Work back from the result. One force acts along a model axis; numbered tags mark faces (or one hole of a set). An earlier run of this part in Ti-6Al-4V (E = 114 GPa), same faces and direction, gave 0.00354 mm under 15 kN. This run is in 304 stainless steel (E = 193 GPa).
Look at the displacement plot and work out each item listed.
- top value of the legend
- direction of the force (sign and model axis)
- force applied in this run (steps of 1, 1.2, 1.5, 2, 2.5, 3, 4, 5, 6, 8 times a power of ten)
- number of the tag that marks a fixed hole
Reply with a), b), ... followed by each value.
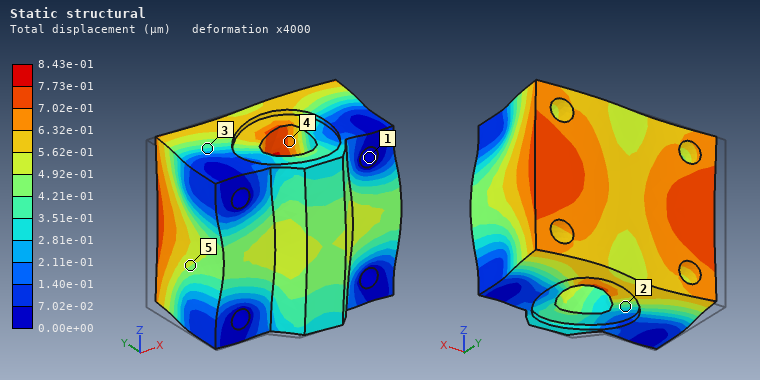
a) 8.43e-01 µm
b) +X
c) 6 kN
d) 1
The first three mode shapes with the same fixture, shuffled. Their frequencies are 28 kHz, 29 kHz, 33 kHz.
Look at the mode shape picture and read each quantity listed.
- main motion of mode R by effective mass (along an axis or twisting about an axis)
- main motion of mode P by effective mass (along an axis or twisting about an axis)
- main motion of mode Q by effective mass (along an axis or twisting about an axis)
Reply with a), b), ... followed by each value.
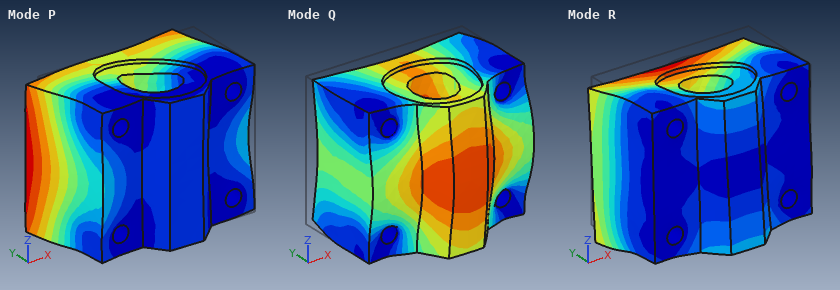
a) along Z
b) along X
c) along Y
